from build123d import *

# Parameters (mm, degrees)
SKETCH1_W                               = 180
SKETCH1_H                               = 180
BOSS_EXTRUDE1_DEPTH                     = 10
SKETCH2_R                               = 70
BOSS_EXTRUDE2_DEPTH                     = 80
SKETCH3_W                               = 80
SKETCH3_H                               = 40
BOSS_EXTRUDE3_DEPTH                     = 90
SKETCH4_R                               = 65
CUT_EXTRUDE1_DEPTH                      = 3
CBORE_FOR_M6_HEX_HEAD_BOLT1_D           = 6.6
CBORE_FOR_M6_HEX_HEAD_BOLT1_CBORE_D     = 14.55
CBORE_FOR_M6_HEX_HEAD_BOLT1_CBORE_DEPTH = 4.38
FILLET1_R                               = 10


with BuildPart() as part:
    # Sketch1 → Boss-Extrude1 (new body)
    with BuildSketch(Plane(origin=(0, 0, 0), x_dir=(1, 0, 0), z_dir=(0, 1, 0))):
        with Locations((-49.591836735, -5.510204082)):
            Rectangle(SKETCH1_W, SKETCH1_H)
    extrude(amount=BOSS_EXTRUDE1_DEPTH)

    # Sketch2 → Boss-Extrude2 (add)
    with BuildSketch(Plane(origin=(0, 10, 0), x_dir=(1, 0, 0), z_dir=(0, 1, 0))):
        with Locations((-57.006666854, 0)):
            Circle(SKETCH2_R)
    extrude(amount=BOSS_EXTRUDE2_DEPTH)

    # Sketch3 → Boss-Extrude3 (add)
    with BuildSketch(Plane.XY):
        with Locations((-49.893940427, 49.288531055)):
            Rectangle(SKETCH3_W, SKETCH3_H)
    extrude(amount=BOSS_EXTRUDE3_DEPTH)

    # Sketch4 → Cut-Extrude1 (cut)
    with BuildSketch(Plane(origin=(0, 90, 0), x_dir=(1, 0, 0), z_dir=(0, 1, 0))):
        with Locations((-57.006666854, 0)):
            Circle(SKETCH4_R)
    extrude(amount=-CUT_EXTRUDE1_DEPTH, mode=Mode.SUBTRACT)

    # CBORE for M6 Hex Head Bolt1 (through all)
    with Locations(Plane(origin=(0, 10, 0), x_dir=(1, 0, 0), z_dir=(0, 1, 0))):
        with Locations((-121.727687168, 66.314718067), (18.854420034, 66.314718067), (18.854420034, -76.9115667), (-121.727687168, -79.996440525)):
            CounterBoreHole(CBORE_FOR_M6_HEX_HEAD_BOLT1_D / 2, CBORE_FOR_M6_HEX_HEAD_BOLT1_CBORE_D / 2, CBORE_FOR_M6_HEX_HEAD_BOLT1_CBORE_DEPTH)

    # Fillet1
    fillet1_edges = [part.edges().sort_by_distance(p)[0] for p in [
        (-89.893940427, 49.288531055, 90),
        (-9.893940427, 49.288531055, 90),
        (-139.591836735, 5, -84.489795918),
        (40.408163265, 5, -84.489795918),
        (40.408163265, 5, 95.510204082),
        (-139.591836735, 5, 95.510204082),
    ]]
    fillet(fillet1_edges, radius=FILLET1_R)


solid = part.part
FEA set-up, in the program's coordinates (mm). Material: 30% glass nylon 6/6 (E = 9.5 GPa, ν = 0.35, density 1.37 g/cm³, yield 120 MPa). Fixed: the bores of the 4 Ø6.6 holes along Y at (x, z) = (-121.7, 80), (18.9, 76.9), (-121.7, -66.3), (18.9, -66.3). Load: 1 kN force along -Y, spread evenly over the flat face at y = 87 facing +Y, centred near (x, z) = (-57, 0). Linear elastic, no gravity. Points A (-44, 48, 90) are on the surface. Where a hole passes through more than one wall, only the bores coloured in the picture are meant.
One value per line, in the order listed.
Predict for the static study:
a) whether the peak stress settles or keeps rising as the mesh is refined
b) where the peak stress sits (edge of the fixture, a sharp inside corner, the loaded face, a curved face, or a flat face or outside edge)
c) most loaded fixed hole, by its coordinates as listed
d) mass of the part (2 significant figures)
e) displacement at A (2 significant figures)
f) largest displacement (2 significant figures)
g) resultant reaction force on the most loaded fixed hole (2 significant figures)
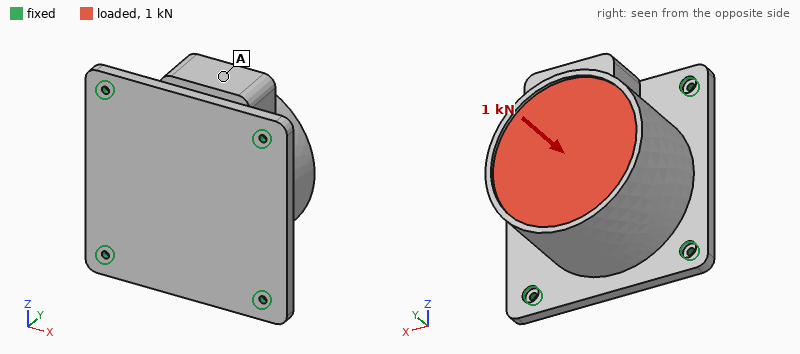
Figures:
keeps rising
edge of the fixture
(-121.7, -66.3)
2.2 kg
59 µm
61 µm
420 N
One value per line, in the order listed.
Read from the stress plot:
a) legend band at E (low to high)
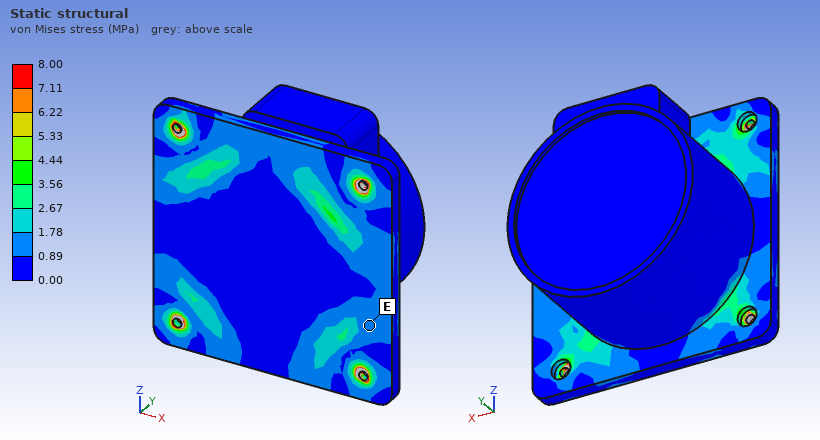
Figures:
0.89 to 1.78 MPa
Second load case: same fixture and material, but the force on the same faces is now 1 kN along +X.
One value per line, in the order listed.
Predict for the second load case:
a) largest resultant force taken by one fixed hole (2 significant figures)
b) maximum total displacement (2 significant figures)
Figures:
600 N
0.11 mm
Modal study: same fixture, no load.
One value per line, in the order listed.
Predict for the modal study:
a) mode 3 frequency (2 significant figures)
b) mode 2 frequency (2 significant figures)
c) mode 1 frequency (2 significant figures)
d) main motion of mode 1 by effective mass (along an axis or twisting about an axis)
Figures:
640 Hz
560 Hz
470 Hz
along Y
